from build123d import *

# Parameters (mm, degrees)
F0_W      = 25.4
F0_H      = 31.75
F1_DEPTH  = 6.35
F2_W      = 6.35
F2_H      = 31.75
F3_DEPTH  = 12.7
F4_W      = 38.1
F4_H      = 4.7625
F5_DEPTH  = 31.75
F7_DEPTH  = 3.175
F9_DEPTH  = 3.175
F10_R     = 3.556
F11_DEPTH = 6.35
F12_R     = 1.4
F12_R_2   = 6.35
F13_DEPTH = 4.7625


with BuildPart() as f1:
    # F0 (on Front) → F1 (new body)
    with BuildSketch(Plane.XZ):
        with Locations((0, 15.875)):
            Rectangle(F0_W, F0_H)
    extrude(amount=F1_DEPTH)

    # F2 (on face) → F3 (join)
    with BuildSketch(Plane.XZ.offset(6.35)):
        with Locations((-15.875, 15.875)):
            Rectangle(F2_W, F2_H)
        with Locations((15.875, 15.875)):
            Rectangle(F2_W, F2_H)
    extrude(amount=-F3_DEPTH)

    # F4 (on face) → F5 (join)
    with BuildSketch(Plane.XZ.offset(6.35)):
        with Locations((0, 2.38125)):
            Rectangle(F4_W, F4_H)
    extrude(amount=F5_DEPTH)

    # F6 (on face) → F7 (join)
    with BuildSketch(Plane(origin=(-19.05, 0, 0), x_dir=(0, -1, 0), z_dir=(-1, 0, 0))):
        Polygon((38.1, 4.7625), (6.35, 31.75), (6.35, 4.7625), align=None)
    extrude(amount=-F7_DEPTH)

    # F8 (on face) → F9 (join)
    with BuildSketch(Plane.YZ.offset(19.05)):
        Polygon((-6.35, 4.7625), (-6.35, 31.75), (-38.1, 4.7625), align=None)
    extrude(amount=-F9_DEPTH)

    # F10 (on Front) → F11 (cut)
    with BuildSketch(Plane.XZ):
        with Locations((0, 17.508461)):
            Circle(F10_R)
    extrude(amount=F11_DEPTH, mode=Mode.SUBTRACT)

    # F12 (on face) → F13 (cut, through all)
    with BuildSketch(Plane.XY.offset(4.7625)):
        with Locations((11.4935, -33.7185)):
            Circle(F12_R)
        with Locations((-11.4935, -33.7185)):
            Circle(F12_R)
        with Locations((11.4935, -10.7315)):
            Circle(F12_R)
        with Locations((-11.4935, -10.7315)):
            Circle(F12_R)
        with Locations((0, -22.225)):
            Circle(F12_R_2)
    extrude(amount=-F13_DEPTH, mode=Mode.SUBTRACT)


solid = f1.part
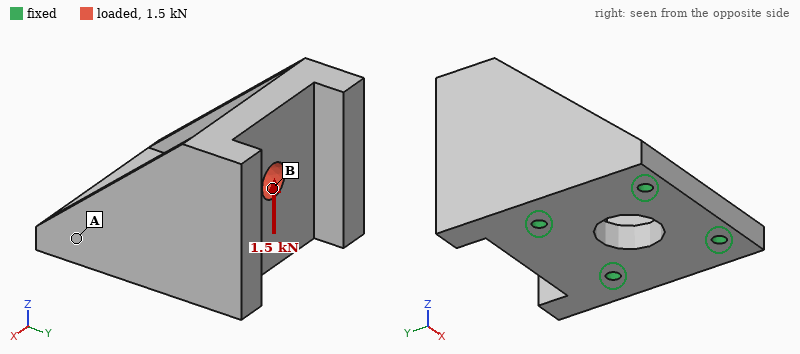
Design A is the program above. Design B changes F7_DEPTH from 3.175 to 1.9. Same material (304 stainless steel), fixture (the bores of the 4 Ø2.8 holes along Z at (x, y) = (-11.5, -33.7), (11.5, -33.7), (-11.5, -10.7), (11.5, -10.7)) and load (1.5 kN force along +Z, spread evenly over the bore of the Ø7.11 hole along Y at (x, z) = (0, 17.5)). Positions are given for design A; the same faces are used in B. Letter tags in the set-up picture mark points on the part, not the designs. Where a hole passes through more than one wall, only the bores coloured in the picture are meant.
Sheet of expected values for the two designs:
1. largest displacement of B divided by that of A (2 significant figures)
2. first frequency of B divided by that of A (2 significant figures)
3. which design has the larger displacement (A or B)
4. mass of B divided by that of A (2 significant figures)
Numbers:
1.1
0.94
B
0.97
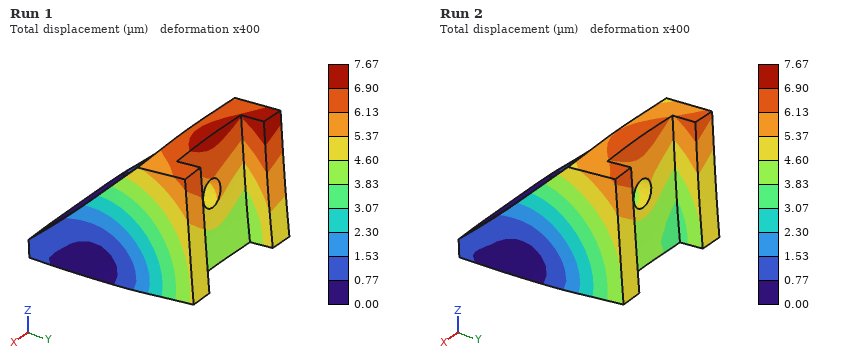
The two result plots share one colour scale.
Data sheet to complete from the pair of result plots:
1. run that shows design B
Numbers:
Run 1
